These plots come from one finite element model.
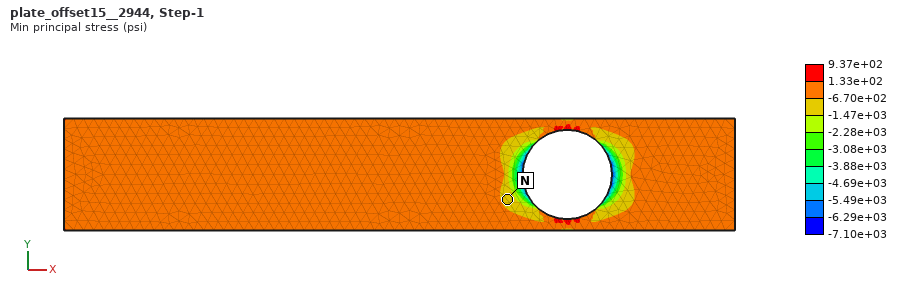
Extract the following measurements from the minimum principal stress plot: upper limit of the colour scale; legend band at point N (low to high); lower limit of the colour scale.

9.37e+02 psi
-1.47e+03 to -6.70e+02 psi
-7.10e+03 psi
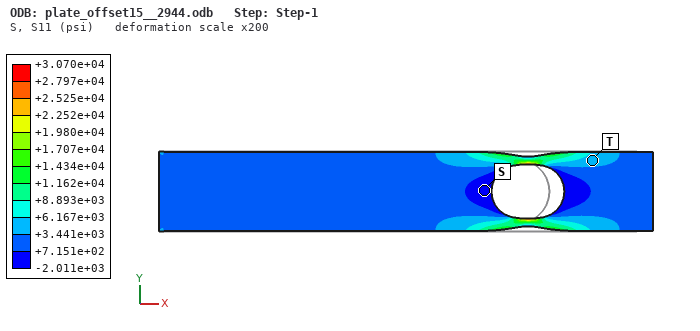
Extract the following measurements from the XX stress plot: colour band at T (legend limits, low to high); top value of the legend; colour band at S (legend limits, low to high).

+3.441e+03 to +6.167e+03 psi
+3.070e+04 psi
-2.011e+03 to +7.151e+02 psi
